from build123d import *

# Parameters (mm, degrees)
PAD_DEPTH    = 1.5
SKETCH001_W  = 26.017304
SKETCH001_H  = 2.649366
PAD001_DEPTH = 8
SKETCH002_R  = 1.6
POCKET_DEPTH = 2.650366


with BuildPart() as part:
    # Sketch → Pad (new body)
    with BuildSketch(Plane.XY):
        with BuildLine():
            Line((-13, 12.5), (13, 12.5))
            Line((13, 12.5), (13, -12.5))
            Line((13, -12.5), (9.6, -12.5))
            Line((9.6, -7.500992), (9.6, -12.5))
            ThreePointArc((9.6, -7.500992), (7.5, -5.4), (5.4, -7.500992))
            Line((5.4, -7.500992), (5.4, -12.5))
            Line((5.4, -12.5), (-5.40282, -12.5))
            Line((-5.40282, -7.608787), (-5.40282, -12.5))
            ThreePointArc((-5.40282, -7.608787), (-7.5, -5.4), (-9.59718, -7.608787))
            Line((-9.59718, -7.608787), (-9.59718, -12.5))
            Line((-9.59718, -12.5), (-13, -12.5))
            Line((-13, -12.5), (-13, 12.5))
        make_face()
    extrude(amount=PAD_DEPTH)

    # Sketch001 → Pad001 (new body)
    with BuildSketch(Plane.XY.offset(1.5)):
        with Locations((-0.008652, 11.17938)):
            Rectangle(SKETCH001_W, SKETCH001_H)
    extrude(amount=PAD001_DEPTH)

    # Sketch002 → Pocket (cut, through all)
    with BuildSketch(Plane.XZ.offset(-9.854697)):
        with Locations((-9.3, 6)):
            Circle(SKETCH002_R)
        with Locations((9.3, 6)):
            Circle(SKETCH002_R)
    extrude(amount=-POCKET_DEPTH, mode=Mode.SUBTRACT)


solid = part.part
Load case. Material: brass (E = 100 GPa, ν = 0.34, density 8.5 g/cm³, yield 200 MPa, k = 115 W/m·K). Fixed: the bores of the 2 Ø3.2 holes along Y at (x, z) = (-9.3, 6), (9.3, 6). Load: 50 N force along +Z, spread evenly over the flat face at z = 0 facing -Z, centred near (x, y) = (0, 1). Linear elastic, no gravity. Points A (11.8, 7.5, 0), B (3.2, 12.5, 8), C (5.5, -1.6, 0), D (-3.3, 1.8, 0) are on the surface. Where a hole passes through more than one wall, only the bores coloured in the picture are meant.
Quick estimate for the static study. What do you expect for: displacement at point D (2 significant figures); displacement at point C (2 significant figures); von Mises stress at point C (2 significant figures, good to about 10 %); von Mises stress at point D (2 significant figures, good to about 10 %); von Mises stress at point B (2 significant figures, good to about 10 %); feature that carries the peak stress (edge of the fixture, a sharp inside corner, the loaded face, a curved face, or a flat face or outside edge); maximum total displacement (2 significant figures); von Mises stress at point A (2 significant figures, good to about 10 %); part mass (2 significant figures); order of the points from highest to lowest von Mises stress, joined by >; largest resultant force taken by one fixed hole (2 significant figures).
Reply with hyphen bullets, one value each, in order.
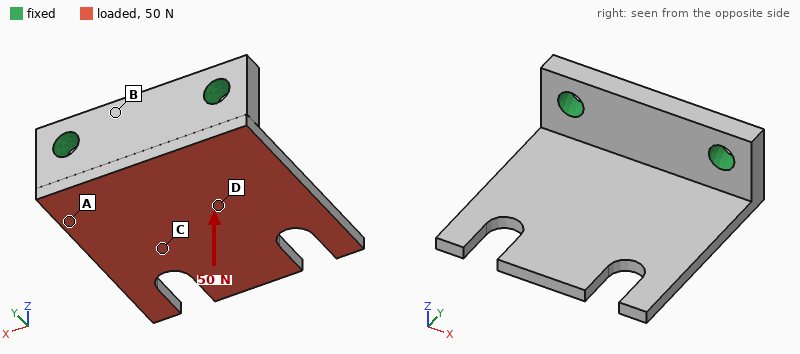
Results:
- 24 µm
- 38 µm
- 9.1 MPa
- 15 MPa
- 4.7 MPa
- the loaded face
- 93 µm
- 35 MPa
- 12 g
- A > D > C > B
- 26 N
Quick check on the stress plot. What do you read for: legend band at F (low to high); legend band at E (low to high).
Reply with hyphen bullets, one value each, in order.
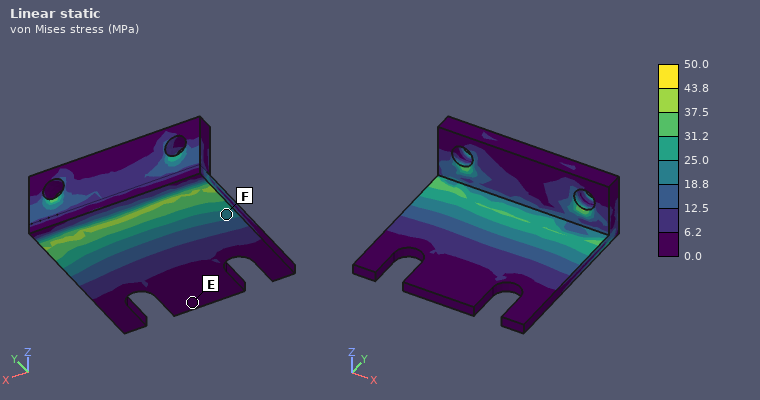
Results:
- 18.8 to 25.0 MPa
- 0.0 to 6.2 MPa
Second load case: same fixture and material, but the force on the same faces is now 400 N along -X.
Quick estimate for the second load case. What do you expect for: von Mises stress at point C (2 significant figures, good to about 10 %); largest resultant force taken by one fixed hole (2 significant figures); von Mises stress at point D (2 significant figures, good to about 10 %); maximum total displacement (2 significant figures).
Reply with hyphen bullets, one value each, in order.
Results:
- 17 MPa
- 310 N
- 20 MPa
- 25 µm
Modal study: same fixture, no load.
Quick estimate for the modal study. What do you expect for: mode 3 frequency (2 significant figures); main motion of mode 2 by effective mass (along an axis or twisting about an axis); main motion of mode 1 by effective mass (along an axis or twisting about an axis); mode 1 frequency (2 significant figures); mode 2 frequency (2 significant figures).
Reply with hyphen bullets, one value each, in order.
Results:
- 6400 Hz
- twisting about Y
- along Z
- 1700 Hz
- 3400 Hz
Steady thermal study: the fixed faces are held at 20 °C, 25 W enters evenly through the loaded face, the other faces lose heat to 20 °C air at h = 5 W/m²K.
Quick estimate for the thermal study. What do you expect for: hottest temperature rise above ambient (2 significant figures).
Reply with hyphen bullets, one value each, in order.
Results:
- 75 K
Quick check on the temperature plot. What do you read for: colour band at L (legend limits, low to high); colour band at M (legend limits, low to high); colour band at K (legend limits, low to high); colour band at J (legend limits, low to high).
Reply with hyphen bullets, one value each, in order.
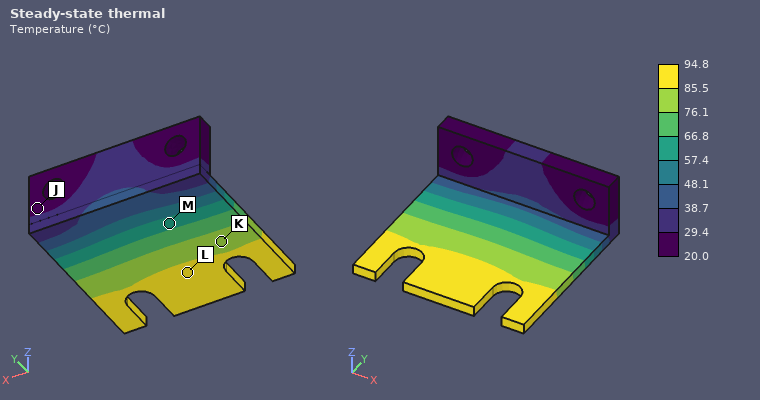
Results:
- 85.5 to 94.8 °C
- 57.4 to 66.8 °C
- 76.1 to 85.5 °C
- 20.0 to 29.4 °C
